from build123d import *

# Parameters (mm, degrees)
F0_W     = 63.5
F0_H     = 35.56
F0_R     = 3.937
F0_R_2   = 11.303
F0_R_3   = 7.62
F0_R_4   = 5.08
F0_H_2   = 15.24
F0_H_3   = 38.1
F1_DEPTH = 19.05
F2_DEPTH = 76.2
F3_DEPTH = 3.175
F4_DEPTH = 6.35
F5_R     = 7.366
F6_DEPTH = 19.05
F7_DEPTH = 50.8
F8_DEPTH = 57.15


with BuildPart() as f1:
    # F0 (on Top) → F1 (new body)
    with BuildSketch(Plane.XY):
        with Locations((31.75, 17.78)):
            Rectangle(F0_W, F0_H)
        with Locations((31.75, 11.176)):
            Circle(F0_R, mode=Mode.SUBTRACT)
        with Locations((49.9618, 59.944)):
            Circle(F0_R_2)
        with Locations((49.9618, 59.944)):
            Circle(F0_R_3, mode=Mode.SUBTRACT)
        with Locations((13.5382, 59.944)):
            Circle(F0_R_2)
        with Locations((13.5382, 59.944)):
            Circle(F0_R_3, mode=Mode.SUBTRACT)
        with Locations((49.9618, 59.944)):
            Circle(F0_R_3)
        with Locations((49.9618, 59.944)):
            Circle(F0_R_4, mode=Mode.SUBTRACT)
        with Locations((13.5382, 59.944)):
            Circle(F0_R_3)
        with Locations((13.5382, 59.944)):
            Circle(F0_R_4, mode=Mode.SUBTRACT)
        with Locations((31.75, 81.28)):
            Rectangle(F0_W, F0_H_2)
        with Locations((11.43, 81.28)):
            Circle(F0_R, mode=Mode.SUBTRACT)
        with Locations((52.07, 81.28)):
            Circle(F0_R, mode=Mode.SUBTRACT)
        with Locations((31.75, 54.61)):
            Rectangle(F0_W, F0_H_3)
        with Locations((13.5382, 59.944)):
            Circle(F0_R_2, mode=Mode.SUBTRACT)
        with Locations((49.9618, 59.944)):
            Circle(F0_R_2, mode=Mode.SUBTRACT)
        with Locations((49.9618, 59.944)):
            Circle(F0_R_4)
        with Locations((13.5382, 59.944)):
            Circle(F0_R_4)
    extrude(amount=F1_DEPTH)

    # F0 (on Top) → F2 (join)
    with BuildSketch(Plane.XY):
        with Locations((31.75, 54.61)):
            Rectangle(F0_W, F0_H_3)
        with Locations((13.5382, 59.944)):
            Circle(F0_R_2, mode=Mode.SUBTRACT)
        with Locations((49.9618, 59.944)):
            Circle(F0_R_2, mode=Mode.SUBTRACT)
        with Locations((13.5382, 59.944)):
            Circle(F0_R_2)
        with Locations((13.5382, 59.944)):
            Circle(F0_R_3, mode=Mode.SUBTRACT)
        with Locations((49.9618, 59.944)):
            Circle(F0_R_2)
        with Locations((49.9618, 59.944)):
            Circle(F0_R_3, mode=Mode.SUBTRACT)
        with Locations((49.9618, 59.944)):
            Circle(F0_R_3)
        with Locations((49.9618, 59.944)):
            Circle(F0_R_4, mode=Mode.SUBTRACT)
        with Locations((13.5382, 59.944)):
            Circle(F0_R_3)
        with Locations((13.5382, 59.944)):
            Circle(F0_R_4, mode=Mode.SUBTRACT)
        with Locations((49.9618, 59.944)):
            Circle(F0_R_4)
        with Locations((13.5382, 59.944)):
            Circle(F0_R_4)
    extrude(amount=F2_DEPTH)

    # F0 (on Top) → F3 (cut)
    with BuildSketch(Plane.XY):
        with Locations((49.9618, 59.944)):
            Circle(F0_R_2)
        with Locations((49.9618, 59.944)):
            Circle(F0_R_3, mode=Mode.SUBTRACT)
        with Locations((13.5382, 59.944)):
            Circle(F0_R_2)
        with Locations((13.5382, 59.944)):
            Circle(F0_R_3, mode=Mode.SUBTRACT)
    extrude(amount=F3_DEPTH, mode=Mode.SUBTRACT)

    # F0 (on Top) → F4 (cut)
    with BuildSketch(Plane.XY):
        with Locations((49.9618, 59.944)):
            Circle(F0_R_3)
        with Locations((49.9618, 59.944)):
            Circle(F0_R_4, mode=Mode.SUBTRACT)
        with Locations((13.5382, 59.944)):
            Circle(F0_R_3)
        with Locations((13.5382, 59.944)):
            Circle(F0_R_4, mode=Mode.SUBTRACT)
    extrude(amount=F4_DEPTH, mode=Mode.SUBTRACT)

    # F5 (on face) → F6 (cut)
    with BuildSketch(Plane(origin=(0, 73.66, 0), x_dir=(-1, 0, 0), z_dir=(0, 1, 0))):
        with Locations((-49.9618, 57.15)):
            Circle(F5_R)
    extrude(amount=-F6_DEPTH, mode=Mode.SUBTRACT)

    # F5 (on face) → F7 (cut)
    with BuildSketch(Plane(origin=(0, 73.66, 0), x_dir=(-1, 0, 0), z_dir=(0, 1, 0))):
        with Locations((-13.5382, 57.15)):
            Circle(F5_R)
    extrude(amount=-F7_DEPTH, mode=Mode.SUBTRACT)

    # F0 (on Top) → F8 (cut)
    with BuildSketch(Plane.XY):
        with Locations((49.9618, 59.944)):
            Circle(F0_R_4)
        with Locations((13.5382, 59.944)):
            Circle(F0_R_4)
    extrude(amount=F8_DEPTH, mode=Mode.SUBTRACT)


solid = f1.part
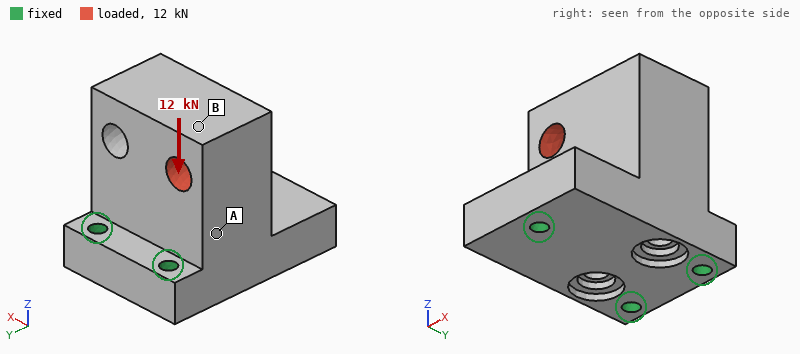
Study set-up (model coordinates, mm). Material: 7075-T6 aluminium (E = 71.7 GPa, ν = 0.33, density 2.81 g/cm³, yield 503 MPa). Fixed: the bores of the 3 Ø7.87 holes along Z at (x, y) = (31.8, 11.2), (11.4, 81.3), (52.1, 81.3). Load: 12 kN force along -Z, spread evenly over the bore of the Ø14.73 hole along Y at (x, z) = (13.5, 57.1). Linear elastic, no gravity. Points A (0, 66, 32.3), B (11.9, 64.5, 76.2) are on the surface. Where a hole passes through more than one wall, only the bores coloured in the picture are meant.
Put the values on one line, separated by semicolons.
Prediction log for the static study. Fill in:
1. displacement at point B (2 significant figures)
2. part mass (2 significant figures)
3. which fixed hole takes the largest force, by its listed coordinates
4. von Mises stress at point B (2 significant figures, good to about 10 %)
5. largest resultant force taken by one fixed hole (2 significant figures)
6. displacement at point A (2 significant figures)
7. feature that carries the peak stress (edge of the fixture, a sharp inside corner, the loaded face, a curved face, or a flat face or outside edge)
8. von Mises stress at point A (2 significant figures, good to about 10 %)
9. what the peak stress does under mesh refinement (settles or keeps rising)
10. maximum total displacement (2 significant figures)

37 µm; 630 g; (11.4, 81.3); 8.5 MPa; 7.9 kN; 21 µm; edge of the fixture; 18 MPa; keeps rising; 43 µm
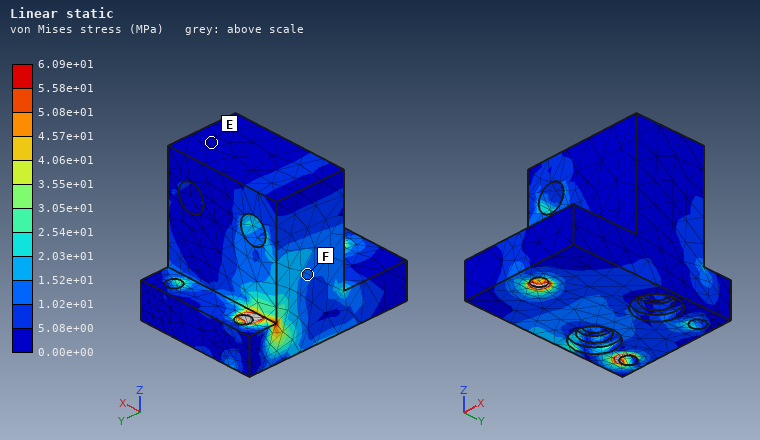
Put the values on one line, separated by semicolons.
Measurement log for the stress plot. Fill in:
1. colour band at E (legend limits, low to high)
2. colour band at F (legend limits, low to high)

0.00e+00 to 5.08e+00 MPa; 1.02e+01 to 1.52e+01 MPa
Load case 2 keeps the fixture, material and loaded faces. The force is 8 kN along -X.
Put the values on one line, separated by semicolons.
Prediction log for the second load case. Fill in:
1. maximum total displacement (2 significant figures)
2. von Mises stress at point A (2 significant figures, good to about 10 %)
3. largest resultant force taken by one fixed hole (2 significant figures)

57 µm; 13 MPa; 7.8 kN
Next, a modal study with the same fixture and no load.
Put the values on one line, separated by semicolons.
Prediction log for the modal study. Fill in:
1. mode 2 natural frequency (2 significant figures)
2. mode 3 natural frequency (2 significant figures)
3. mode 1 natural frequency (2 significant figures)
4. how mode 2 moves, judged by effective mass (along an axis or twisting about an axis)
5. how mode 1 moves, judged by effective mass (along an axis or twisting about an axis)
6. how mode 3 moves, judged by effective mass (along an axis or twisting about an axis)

4400 Hz; 8900 Hz; 4100 Hz; along Y; along X; along Z
